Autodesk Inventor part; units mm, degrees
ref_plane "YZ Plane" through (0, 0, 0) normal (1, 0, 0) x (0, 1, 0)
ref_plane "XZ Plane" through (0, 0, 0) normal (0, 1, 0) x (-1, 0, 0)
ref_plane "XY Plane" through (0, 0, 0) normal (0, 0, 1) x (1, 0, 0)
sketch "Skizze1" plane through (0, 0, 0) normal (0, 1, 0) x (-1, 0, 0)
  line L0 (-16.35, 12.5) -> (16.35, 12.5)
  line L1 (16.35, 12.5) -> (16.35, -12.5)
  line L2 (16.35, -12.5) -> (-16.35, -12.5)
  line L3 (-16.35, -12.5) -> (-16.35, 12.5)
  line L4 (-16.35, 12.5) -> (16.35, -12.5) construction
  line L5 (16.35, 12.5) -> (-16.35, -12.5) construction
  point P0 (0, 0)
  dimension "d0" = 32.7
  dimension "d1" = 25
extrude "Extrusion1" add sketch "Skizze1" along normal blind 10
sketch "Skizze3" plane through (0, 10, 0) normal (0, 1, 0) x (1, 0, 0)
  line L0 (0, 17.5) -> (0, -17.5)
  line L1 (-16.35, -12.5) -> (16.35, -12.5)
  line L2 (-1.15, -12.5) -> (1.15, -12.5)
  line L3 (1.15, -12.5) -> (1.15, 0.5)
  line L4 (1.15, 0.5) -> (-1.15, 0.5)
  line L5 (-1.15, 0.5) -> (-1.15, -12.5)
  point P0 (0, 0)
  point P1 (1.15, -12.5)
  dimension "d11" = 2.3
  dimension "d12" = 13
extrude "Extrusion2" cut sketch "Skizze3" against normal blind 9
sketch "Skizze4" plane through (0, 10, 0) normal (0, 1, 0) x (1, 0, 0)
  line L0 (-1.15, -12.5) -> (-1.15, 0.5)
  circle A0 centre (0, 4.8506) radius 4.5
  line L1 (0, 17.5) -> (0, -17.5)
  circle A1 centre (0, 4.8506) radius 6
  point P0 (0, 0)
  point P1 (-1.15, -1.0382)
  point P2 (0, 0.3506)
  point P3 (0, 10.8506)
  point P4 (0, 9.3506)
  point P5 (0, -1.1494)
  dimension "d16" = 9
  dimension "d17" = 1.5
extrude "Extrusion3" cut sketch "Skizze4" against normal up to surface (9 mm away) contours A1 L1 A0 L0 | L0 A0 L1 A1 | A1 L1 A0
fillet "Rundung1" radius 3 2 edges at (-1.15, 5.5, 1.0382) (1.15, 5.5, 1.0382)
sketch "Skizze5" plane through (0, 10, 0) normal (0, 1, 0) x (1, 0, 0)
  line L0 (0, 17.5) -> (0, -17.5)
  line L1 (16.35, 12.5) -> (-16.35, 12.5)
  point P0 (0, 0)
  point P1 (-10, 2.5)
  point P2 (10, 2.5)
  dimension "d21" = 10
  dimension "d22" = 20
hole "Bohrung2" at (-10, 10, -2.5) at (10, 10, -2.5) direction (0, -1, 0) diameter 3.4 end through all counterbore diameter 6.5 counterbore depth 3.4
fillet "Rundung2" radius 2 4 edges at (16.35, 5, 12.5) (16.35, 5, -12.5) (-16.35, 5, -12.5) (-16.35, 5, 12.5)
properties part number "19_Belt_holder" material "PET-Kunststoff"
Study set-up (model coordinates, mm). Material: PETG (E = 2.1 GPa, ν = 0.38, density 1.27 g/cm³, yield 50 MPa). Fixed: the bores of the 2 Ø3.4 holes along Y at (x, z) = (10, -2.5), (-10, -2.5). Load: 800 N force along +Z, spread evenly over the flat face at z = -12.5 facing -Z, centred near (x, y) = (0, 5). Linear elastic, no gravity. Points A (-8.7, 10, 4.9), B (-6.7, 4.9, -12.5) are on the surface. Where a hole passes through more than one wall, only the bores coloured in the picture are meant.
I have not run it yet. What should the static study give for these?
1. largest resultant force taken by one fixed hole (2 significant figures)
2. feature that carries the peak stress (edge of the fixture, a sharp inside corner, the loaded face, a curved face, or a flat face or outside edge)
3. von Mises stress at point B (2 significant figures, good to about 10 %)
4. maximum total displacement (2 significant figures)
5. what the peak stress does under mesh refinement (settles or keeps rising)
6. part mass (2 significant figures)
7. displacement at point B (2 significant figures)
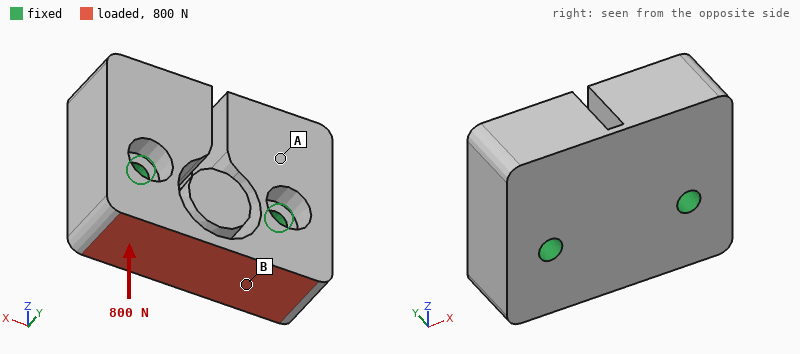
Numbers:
410 N
edge of the fixture
5.6 MPa
0.14 mm
keeps rising
9.0 g
0.054 mm
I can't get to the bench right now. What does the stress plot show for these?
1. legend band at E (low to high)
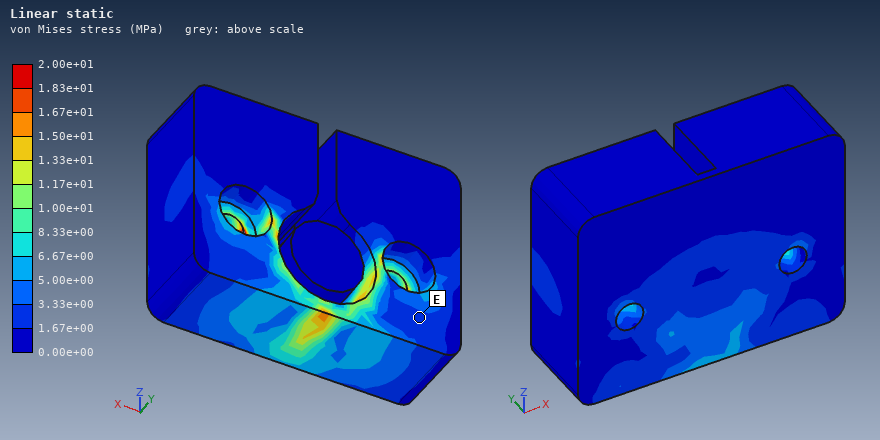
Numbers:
1.67e+00 to 3.33e+00 MPa
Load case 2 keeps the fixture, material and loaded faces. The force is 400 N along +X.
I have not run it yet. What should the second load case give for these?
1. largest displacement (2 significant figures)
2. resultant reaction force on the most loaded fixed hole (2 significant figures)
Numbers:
74 µm
240 N
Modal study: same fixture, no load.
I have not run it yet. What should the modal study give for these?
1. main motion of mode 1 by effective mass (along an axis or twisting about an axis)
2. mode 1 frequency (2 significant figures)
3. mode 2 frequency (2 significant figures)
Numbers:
along Y
4300 Hz
4900 Hz
